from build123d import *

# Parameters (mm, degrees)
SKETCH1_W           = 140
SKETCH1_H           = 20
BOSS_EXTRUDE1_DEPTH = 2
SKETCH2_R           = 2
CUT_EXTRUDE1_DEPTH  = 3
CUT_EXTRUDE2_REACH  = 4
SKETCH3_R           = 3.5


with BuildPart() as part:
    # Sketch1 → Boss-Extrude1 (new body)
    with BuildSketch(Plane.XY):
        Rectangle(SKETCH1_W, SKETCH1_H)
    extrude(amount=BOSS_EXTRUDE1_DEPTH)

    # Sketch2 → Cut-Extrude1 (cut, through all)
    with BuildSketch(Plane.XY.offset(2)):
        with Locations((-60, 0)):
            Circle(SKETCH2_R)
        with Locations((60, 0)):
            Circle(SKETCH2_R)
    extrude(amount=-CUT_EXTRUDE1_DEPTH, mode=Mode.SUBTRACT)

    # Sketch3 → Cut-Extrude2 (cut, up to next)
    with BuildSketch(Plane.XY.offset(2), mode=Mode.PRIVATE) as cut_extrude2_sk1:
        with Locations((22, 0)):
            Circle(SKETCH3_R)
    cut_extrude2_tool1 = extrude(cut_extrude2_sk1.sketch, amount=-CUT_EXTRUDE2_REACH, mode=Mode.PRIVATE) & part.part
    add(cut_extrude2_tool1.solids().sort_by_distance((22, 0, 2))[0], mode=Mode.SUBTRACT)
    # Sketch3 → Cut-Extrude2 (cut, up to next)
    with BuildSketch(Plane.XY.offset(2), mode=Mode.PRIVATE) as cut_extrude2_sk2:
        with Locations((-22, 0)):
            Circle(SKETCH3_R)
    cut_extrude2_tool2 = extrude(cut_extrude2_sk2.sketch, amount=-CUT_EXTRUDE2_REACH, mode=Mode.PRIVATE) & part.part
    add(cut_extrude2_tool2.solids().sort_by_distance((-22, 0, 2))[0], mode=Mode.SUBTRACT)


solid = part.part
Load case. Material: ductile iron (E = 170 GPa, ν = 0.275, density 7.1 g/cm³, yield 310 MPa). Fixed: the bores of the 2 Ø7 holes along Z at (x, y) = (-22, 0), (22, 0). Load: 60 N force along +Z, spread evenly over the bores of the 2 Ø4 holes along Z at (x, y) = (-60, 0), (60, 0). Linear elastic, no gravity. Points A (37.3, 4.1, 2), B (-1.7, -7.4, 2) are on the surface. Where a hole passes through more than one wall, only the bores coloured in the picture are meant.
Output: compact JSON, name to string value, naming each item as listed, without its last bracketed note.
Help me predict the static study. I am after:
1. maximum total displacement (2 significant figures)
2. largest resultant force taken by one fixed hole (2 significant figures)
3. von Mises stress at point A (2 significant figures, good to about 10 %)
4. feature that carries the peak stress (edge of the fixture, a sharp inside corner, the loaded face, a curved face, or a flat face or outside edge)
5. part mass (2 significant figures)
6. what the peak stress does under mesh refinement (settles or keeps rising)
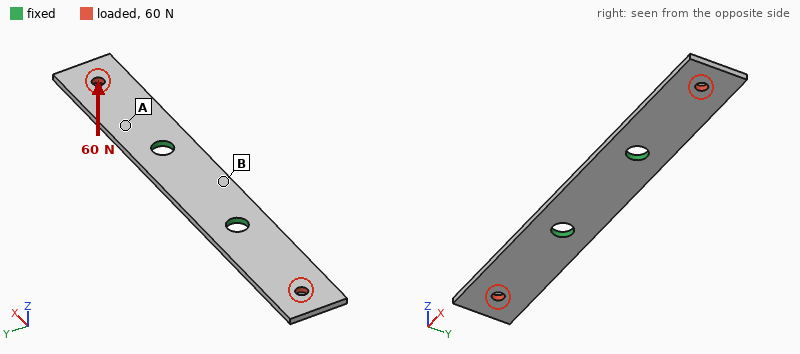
{"maximum total displacement": "0.28 mm", "largest resultant force taken by one fixed hole": "30 N", "von Mises stress at point A": "48 MPa", "feature that carries the peak stress": "edge of the fixture", "part mass": "38 g", "what the peak stress does under mesh refinement": "keeps rising"}
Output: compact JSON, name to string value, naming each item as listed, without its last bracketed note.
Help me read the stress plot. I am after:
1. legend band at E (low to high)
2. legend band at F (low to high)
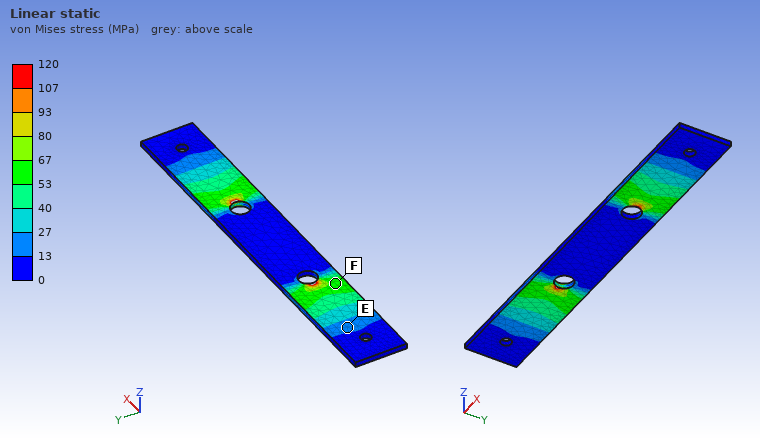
{"legend band at E": "13 to 27 MPa", "legend band at F": "53 to 67 MPa"}
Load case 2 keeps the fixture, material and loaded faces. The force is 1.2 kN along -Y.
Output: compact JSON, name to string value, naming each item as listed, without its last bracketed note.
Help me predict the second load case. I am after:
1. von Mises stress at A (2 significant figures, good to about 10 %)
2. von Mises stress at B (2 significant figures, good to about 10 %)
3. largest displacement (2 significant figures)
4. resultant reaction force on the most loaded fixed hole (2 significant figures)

{"von Mises stress at A": "53 MPa", "von Mises stress at B": "33 MPa", "largest displacement": "0.11 mm", "resultant reaction force on the most loaded fixed hole": "600 N"}
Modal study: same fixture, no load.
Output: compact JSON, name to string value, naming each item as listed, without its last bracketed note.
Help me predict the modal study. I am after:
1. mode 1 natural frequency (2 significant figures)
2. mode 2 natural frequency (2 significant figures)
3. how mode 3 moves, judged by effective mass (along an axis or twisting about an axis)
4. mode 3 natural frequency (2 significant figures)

{"mode 1 natural frequency": "780 Hz", "mode 2 natural frequency": "780 Hz", "how mode 3 moves, judged by effective mass": "twisting about X", "mode 3 natural frequency": "3400 Hz"}
